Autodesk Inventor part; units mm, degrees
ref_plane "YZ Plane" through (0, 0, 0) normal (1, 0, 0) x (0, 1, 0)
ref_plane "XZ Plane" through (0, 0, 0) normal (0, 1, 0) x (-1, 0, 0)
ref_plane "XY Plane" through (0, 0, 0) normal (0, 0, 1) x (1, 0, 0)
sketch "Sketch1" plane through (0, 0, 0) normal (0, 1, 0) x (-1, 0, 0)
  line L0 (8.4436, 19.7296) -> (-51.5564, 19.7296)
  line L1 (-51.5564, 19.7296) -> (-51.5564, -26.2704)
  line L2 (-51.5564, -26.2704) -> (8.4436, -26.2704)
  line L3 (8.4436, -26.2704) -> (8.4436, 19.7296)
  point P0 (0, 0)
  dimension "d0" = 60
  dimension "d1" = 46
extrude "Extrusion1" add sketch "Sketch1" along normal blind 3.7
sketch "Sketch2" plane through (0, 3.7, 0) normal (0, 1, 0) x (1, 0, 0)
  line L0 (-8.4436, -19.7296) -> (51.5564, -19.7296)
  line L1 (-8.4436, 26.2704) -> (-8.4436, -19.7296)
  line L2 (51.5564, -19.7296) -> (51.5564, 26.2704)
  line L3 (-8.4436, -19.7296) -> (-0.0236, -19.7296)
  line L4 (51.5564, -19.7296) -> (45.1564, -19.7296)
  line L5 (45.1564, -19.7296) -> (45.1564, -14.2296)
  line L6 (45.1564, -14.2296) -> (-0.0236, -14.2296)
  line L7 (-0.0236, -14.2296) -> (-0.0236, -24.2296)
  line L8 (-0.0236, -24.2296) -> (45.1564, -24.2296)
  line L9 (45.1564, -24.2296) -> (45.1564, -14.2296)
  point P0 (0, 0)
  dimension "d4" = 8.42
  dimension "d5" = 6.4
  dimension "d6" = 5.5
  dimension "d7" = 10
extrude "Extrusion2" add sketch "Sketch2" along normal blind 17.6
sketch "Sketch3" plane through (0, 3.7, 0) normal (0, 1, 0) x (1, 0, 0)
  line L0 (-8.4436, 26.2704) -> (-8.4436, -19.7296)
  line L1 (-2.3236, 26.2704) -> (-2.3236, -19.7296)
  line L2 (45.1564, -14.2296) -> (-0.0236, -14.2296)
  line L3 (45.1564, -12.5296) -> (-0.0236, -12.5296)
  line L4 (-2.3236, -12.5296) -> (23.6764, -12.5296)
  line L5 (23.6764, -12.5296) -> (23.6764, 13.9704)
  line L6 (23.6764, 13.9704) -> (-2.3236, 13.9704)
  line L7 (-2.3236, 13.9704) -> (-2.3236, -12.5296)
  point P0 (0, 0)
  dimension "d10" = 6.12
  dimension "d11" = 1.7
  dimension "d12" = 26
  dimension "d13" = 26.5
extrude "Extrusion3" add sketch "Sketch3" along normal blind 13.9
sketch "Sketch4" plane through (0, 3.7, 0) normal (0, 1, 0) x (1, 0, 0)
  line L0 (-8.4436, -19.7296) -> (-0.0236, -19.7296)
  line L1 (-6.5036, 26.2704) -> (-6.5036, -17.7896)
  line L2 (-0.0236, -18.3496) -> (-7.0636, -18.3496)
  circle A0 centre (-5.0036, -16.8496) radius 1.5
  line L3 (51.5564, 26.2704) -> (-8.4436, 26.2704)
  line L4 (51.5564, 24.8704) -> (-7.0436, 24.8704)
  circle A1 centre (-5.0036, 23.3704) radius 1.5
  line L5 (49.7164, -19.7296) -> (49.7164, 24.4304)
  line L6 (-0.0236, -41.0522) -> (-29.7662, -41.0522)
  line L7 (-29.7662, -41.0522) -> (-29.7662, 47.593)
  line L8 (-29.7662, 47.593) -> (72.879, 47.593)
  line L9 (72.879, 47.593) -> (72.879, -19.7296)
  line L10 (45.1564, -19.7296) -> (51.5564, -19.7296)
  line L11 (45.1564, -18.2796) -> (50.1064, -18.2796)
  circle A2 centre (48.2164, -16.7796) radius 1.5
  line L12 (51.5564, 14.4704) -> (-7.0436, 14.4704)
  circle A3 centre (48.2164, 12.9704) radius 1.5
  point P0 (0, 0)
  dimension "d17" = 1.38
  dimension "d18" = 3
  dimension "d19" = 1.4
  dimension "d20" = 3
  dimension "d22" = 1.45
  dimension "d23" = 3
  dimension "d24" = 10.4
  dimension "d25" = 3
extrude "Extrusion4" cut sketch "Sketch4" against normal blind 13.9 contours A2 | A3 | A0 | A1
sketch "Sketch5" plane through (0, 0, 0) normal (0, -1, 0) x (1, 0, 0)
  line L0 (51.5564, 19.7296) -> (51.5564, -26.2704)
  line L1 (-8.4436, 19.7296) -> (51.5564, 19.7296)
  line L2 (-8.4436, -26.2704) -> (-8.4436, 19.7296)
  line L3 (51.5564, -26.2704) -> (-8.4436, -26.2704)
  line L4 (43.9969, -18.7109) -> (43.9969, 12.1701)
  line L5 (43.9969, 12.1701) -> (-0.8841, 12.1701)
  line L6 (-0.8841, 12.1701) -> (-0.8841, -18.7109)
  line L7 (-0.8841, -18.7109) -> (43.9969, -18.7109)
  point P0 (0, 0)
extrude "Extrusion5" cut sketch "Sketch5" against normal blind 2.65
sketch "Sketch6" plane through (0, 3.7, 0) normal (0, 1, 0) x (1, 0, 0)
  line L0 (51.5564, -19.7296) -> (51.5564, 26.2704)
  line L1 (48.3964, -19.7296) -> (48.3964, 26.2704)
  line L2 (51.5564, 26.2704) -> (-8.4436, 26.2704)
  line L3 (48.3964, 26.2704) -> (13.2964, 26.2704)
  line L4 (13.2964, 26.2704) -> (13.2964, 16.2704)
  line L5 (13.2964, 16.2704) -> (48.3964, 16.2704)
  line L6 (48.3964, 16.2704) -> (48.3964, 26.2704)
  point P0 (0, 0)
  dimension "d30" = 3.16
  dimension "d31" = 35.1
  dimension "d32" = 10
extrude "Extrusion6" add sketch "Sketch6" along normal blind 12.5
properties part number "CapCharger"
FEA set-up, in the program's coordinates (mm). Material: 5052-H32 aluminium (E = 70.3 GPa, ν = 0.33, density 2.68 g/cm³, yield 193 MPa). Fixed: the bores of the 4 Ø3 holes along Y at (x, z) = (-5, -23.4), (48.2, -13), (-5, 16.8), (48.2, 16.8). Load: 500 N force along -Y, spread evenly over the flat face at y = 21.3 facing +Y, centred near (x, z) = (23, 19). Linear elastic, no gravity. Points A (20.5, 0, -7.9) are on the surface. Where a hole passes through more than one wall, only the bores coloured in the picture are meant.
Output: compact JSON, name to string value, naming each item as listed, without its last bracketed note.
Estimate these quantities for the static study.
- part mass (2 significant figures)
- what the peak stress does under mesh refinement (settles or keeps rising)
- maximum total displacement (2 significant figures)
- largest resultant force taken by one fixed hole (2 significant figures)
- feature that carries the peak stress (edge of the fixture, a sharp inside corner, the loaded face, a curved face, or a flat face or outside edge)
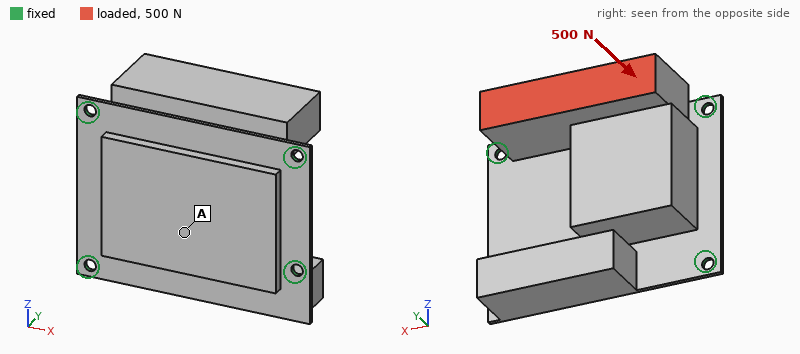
{"part mass": "76 g", "what the peak stress does under mesh refinement": "keeps rising", "maximum total displacement": "0.12 mm", "largest resultant force taken by one fixed hole": "330 N", "feature that carries the peak stress": "edge of the fixture"}
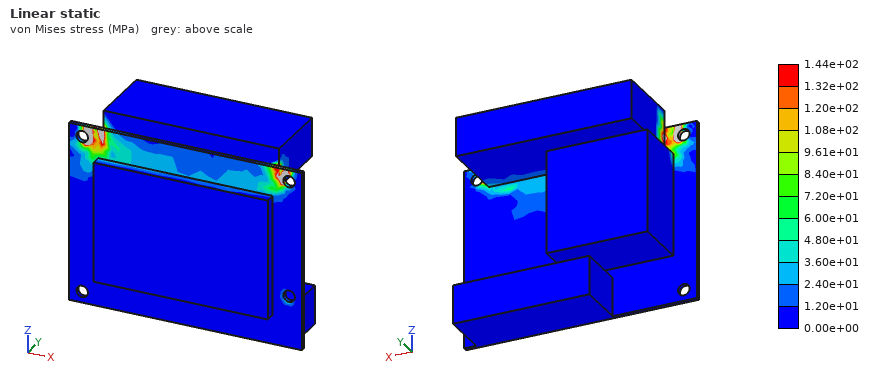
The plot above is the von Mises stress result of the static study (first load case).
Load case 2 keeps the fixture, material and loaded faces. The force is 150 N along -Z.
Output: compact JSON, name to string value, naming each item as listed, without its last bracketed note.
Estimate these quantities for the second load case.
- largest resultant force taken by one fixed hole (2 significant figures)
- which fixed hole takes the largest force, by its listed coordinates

{"largest resultant force taken by one fixed hole": "96 N", "which fixed hole takes the largest force, by its listed coordinates": "(48.2, 16.8)"}
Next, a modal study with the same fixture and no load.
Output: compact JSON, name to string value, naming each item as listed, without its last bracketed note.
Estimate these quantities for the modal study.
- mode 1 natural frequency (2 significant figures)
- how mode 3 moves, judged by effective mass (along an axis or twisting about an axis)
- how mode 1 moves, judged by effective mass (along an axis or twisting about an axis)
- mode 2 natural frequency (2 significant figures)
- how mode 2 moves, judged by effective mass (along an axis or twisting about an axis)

{"mode 1 natural frequency": "1600 Hz", "how mode 3 moves, judged by effective mass": "along Y", "how mode 1 moves, judged by effective mass": "along Z", "mode 2 natural frequency": "2300 Hz", "how mode 2 moves, judged by effective mass": "along Y"}
